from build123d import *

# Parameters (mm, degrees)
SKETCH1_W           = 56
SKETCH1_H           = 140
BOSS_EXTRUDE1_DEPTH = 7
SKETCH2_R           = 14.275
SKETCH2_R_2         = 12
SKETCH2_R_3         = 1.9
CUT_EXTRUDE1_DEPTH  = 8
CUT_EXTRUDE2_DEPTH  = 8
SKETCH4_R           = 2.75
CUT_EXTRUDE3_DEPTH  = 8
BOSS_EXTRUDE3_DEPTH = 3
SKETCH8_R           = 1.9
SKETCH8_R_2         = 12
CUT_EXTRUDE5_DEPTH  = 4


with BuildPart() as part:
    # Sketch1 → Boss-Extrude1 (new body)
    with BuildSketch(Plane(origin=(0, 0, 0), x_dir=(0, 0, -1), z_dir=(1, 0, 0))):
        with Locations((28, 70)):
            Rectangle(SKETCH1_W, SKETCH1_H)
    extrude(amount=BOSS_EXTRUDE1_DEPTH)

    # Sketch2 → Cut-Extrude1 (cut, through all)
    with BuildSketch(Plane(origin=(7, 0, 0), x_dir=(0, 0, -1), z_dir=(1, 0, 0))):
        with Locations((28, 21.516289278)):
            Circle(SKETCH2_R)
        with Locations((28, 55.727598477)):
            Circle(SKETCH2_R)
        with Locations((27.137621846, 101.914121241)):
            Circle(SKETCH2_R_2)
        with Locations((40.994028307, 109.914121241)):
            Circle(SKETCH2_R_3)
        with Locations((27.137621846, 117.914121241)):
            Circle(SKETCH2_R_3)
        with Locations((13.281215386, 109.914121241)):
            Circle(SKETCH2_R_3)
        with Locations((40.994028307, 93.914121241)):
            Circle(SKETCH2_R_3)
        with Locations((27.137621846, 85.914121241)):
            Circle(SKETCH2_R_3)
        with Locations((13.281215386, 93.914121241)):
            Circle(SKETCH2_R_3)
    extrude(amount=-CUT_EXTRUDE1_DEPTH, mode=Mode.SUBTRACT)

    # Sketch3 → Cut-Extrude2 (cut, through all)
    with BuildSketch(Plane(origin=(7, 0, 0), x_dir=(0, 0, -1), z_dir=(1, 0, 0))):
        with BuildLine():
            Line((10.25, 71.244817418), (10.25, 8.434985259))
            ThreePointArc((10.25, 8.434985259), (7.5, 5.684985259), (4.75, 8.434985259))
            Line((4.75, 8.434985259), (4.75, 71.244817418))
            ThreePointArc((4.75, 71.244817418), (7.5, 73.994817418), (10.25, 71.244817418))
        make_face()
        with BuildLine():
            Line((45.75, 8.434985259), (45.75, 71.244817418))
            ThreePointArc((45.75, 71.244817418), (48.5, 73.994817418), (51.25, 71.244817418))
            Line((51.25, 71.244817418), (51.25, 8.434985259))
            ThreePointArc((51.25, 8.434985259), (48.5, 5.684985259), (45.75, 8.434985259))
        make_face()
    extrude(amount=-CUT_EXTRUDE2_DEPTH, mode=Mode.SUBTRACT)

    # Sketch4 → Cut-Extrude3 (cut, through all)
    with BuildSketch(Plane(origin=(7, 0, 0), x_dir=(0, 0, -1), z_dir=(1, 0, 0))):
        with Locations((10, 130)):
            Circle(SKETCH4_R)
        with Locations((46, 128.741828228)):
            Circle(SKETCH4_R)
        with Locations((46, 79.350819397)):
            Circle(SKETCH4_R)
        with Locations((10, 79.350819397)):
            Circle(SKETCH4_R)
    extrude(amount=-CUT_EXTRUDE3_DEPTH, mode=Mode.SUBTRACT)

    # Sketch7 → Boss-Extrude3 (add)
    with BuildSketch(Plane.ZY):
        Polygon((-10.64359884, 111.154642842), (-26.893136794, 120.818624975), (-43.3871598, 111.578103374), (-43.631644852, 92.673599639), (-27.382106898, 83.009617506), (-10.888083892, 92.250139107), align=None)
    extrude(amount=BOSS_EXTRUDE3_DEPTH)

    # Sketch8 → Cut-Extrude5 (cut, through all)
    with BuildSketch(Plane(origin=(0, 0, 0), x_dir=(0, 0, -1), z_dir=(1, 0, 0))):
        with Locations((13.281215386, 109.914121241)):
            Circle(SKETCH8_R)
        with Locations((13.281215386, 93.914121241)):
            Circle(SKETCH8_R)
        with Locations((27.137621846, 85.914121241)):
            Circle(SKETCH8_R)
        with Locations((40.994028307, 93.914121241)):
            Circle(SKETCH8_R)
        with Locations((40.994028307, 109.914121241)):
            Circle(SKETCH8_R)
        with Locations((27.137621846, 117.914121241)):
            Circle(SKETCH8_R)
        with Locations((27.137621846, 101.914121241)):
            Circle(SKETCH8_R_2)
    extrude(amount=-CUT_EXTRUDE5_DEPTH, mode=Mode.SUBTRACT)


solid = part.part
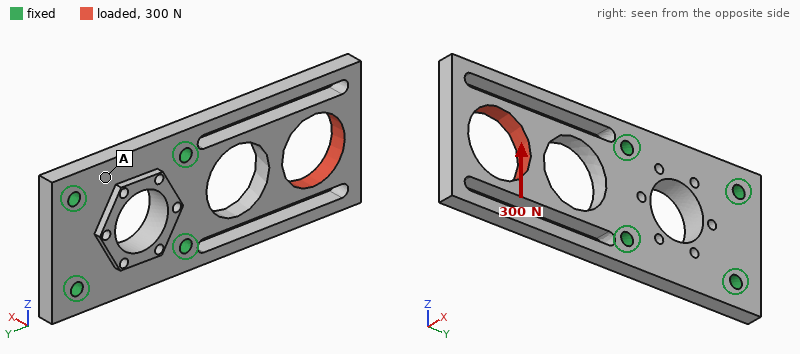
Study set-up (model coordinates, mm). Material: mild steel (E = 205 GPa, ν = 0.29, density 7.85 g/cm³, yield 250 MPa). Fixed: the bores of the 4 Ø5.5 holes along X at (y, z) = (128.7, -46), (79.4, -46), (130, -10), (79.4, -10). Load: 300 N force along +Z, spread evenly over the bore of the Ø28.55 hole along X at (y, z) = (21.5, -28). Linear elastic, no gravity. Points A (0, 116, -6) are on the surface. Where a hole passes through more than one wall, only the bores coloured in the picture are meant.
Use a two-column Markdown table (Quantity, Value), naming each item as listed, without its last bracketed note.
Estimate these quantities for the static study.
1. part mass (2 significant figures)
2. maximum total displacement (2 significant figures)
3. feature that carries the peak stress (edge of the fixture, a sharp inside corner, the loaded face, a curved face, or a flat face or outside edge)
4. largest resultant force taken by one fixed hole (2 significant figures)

| Quantity | Value |
|---|---|
| part mass | 300 g |
| maximum total displacement | 23 µm |
| feature that carries the peak stress | a flat face or outside edge |
| largest resultant force taken by one fixed hole | 440 N |
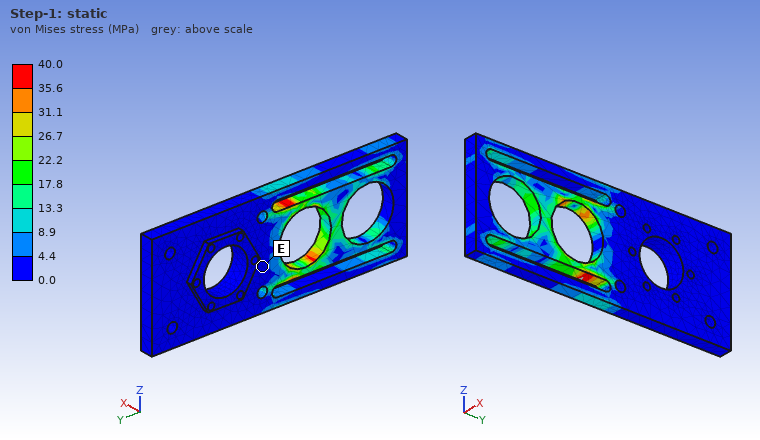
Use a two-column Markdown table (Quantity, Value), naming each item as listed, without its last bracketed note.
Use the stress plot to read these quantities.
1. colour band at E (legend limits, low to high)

| Quantity | Value |
|---|---|
| colour band at E | 0.0 to 4.4 MPa |
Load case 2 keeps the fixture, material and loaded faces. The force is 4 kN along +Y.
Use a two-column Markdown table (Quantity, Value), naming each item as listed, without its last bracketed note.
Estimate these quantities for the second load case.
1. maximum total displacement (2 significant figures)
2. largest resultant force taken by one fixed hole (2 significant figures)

| Quantity | Value |
|---|---|
| maximum total displacement | 22 µm |
| largest resultant force taken by one fixed hole | 1.9 kN |
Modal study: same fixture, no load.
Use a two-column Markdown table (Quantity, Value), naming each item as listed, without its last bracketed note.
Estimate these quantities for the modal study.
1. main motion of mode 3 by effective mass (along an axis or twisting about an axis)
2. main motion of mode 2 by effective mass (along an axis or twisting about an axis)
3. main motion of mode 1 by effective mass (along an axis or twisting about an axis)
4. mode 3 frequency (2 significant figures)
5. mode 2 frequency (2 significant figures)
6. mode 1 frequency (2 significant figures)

| Quantity | Value |
|---|---|
| main motion of mode 3 by effective mass | along Z |
| main motion of mode 2 by effective mass | twisting about Y |
| main motion of mode 1 by effective mass | along X |
| mode 3 frequency | 2200 Hz |
| mode 2 frequency | 1800 Hz |
| mode 1 frequency | 760 Hz |
